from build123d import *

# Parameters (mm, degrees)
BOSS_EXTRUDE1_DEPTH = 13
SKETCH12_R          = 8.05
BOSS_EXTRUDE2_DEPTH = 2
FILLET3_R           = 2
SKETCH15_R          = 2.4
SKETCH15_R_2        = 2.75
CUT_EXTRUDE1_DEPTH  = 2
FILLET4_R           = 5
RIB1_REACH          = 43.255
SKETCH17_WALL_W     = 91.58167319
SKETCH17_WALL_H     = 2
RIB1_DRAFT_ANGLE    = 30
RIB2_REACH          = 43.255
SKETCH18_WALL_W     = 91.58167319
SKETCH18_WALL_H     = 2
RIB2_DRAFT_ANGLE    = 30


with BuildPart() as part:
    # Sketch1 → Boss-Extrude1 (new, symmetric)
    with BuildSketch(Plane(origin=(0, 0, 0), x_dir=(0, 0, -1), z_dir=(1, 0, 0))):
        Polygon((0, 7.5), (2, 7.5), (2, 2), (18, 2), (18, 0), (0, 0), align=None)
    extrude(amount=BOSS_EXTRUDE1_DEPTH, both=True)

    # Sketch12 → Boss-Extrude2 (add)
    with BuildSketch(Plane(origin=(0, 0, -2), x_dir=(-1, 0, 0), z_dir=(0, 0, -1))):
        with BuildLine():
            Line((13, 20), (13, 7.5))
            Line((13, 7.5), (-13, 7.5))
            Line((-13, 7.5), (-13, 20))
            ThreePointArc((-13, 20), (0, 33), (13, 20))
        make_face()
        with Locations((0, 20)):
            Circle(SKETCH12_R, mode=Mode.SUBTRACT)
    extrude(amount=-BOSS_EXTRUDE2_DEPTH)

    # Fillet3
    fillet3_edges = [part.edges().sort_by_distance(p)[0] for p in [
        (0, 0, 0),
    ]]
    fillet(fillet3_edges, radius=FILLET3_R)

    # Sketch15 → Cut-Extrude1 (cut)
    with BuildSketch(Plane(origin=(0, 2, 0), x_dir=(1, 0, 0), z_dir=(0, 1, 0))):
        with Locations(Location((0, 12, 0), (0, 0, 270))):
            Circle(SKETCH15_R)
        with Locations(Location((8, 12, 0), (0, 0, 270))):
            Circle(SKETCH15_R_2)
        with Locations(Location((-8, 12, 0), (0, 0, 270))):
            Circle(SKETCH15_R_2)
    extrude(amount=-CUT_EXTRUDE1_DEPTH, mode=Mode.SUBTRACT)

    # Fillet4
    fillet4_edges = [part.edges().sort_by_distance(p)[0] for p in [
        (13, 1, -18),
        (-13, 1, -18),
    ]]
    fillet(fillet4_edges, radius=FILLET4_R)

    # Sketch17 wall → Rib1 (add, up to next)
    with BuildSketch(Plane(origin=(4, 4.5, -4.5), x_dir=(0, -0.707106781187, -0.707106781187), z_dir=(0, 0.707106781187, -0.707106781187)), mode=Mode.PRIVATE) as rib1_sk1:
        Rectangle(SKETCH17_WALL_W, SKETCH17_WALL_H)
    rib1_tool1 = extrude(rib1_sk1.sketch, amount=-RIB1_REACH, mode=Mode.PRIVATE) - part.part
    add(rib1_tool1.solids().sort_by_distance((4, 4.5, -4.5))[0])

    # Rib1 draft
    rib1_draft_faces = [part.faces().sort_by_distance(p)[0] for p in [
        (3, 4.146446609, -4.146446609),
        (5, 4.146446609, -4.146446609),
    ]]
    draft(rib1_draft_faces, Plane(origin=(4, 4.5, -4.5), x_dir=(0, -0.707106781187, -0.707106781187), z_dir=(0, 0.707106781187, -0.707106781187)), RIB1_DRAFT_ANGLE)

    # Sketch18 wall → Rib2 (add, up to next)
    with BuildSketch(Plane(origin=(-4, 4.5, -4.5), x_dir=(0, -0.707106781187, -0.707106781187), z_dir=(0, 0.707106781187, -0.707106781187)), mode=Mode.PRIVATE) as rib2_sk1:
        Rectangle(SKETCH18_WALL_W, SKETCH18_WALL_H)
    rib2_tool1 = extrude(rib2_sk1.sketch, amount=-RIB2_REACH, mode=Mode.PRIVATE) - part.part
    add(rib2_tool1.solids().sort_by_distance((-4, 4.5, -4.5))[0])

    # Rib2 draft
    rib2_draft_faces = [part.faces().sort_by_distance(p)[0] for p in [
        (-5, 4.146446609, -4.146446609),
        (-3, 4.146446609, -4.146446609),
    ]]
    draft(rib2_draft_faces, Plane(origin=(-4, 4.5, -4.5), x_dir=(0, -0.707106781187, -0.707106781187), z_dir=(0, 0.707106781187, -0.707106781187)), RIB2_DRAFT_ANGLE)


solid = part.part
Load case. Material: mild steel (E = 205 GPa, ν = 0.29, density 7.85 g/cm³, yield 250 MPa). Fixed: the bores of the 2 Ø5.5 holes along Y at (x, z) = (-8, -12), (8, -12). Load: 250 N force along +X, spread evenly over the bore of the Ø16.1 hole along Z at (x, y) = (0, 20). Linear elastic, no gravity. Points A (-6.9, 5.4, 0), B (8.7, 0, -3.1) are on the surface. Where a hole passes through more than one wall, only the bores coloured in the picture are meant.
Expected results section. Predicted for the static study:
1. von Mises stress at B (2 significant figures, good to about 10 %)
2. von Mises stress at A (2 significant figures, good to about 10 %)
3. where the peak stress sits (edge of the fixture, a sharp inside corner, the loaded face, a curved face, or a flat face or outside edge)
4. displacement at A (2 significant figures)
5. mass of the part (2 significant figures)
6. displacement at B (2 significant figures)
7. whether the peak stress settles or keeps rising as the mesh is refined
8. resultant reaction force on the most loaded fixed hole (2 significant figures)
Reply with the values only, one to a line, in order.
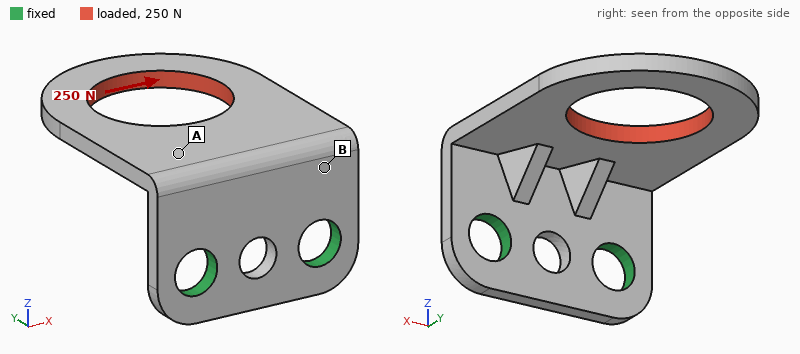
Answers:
73 MPa
25 MPa
edge of the fixture
14 µm
15 g
11 µm
keeps rising
340 N
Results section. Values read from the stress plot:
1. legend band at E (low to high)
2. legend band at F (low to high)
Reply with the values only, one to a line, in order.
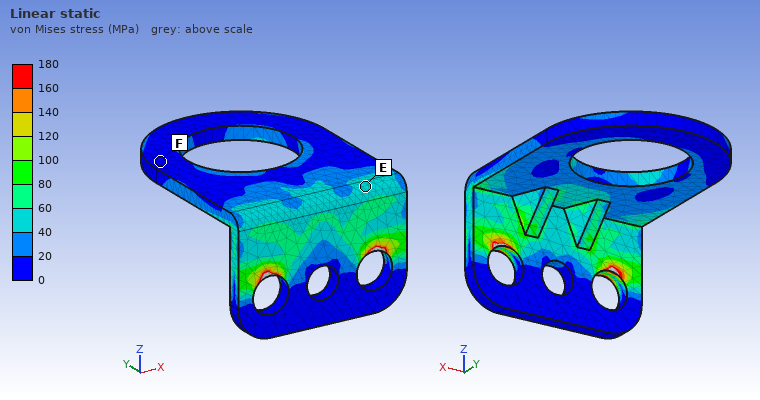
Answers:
40 to 60 MPa
0 to 20 MPa
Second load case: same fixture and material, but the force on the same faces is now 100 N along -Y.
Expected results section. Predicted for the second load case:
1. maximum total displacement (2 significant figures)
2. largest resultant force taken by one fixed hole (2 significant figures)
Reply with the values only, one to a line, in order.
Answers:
32 µm
50 N
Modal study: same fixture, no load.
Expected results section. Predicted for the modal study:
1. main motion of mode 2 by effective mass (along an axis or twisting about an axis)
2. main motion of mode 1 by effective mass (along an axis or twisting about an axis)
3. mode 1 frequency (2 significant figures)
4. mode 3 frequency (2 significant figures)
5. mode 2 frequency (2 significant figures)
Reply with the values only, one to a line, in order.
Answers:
along X
along Z
1800 Hz
5700 Hz
4400 Hz
